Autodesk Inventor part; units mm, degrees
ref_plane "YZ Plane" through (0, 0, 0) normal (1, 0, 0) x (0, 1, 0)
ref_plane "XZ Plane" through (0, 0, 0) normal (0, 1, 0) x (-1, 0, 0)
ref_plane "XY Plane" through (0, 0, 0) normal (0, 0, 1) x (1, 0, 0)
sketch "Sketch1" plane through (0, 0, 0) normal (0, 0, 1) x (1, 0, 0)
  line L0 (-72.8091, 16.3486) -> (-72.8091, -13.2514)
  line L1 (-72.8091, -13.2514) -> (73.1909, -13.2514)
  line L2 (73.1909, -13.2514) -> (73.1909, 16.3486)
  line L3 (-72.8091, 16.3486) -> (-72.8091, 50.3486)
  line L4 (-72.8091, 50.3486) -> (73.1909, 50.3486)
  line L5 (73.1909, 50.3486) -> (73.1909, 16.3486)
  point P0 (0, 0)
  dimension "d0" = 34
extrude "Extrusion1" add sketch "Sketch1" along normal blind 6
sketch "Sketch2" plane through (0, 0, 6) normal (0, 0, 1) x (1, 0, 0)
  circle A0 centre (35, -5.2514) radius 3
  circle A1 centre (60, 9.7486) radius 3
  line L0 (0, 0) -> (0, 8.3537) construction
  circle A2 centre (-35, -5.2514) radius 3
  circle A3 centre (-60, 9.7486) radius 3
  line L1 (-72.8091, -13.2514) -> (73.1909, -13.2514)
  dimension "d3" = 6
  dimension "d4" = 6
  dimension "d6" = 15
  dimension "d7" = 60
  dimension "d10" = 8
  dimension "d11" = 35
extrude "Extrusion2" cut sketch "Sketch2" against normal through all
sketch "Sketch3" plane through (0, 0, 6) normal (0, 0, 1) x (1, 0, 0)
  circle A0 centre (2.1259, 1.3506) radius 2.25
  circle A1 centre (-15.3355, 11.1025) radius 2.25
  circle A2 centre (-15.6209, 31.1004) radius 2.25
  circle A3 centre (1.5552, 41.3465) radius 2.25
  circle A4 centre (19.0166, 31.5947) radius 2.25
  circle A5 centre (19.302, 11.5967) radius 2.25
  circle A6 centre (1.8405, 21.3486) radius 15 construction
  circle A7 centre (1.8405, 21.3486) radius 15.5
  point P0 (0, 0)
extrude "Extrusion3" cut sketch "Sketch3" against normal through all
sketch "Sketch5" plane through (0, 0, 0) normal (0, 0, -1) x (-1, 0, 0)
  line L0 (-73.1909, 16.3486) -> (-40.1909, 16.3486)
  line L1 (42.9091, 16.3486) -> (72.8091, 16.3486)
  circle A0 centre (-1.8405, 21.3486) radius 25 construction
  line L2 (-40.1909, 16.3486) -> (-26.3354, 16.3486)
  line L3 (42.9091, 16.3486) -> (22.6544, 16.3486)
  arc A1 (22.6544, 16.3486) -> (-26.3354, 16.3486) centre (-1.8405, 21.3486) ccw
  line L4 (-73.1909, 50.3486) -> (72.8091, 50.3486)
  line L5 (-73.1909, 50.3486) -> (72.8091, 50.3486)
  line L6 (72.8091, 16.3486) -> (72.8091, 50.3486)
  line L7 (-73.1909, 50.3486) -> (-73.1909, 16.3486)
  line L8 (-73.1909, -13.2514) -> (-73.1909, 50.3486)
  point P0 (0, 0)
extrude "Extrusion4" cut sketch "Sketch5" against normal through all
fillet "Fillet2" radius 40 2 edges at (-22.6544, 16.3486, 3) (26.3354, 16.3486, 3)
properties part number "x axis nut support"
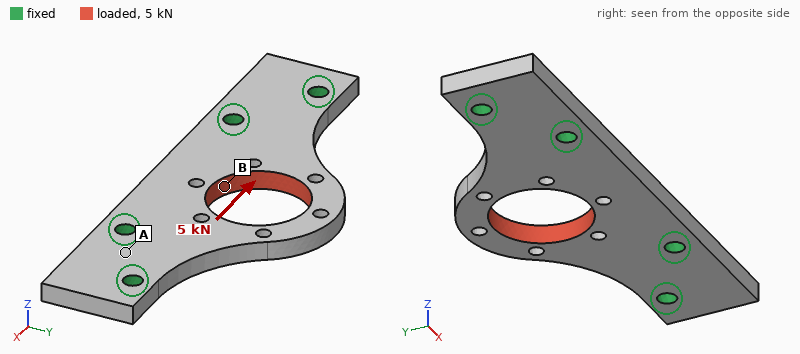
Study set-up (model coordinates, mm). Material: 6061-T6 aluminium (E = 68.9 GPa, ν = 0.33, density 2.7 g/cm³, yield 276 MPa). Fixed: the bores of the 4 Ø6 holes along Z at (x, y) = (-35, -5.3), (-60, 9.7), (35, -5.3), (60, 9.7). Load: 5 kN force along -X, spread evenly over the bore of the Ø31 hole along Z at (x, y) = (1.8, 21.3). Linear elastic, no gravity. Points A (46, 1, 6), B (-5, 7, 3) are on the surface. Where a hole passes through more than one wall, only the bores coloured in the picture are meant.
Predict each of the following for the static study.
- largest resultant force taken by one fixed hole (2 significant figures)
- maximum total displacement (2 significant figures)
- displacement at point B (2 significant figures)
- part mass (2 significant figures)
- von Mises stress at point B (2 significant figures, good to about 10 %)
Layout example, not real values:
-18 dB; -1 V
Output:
1.5 kN; 40 µm; 6.4 µm; 79 g; 21 MPa
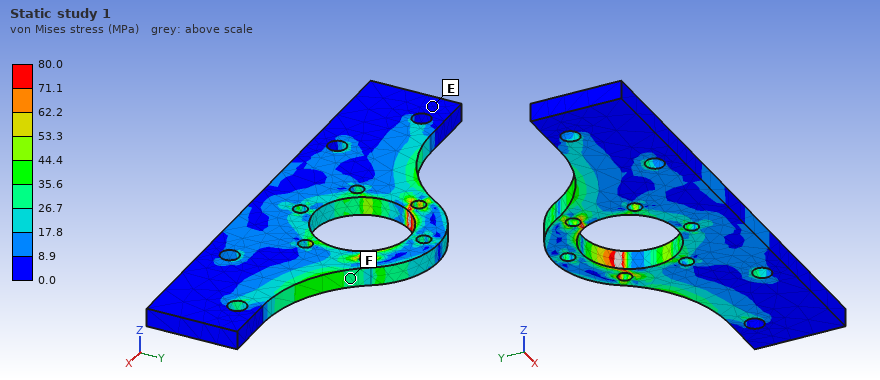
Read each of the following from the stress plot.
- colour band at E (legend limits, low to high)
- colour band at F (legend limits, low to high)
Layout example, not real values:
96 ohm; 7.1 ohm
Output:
0.0 to 8.9 MPa; 26.7 to 35.6 MPa
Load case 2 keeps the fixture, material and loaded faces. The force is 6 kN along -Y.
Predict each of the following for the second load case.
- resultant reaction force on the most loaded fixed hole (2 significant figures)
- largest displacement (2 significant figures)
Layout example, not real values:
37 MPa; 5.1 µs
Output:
3.5 kN; 29 µm
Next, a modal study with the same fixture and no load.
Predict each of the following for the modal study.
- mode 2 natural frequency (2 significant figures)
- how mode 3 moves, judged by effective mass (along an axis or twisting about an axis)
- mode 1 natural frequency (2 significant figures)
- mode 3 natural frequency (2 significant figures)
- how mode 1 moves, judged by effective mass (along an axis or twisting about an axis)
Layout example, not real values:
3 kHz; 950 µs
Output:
6000 Hz; along Z; 2500 Hz; 6700 Hz; along Z
